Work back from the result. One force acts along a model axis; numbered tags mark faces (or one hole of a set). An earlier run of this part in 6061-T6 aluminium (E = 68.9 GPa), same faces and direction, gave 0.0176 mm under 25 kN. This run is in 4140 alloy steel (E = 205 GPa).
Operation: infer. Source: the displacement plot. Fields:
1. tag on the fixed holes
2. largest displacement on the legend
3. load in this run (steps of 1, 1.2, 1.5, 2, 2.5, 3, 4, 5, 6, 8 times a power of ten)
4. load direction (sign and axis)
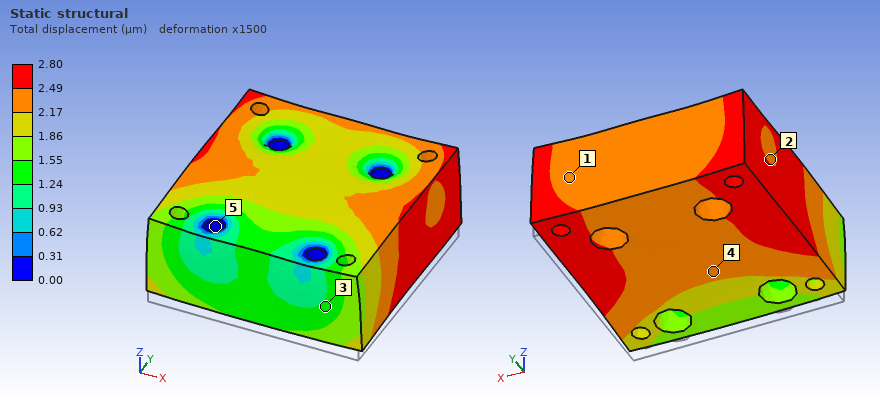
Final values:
5
2.80 µm
12 kN
+Z
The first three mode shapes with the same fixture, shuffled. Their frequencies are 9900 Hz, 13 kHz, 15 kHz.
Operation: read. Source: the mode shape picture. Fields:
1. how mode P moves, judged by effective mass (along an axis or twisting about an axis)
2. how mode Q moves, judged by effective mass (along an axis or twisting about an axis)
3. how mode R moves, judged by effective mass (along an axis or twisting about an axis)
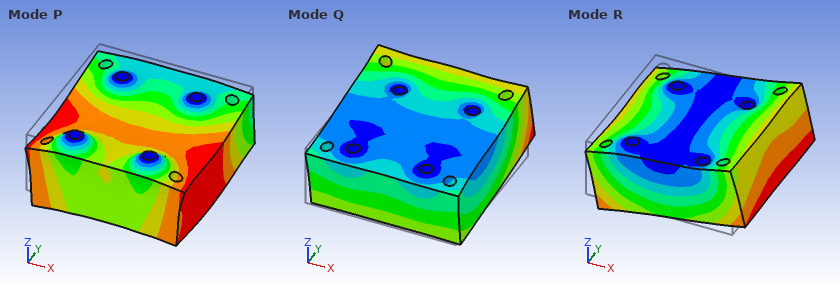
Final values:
along Z
along Y
along X
